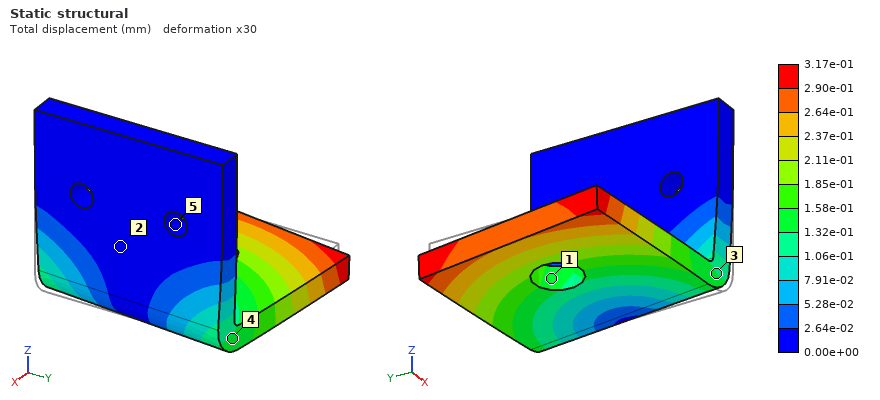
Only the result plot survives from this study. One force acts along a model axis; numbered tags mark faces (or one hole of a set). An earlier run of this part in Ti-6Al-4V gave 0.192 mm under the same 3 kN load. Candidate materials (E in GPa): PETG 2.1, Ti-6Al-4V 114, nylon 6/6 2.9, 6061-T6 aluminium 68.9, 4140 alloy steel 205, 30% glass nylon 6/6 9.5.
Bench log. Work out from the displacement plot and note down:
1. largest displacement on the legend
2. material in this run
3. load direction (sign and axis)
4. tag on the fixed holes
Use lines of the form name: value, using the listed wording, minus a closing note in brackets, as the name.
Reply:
largest displacement on the legend: 3.17e-01 mm
material in this run: 6061-T6 aluminium
load direction: +Y
tag on the fixed holes: 5
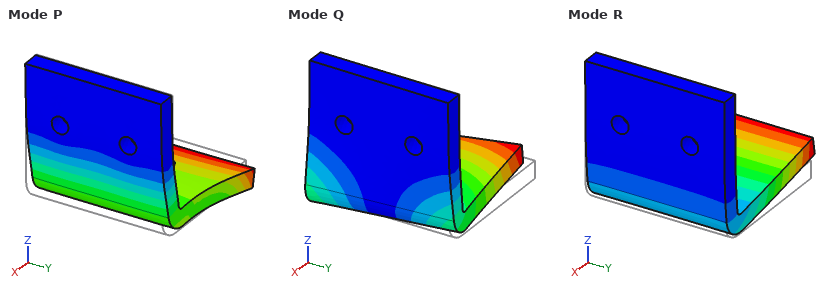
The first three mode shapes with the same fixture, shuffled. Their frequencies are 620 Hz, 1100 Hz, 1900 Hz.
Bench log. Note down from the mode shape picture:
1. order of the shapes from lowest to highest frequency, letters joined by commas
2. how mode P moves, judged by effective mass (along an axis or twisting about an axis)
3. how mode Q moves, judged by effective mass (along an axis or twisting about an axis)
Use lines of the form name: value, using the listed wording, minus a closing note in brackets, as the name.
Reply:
order of the shapes from lowest to highest frequency, letters joined by commas: R, Q, P
how mode P moves, judged by effective mass: along X
how mode Q moves, judged by effective mass: along Y
